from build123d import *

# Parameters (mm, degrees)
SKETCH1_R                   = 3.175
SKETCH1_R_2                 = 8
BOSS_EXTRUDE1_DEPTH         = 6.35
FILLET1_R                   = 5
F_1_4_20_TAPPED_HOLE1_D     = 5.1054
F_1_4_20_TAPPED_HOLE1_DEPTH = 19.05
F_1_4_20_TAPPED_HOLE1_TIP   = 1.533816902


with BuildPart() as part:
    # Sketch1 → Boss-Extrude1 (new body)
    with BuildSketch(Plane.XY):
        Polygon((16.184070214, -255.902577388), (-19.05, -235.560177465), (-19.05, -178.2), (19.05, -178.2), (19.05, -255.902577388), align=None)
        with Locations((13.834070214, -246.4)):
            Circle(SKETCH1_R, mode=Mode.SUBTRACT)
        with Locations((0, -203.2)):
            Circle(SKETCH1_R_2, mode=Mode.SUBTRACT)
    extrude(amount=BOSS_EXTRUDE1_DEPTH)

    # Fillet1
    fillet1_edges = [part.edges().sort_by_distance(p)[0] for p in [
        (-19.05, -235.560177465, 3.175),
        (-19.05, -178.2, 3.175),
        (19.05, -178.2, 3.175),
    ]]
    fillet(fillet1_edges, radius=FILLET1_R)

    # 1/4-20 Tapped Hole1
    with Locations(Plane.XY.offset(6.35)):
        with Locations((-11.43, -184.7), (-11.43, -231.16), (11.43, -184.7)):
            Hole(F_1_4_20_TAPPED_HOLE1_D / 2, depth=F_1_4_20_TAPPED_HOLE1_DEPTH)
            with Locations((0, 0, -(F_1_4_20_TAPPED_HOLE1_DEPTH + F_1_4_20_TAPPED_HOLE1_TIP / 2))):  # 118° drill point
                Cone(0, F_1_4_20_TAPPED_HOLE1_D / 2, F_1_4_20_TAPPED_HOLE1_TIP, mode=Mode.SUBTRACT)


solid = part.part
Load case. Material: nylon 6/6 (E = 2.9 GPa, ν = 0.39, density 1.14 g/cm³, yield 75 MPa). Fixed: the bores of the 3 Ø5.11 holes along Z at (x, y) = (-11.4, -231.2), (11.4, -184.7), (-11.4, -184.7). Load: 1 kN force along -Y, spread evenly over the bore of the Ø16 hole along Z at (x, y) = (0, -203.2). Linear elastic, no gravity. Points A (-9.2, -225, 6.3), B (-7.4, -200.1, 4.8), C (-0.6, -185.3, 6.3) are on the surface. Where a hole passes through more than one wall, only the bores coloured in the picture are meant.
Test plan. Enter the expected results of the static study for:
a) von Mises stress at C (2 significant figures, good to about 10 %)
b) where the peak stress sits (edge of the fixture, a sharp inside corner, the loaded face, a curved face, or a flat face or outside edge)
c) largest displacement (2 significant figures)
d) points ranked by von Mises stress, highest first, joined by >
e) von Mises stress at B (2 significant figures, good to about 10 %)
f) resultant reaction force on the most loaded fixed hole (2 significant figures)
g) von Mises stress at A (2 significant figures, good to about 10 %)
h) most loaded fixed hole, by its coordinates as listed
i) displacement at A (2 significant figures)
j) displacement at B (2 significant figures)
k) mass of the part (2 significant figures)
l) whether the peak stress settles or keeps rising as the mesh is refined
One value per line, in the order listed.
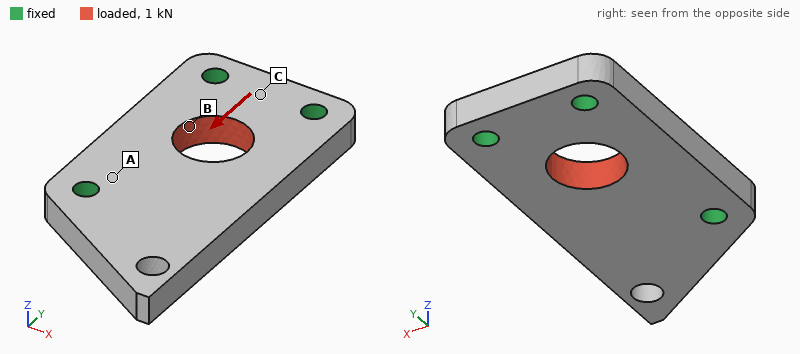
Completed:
1.1 MPa
edge of the fixture
41 µm
B > A > C
5.3 MPa
390 N
3.8 MPa
(11.4, -184.7)
7.3 µm
20 µm
17 g
keeps rising
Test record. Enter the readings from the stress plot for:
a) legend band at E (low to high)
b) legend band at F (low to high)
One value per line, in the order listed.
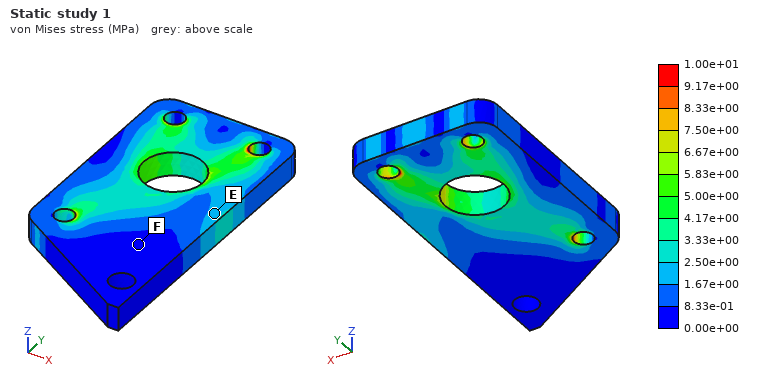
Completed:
1.67e+00 to 2.50e+00 MPa
0.00e+00 to 8.33e-01 MPa
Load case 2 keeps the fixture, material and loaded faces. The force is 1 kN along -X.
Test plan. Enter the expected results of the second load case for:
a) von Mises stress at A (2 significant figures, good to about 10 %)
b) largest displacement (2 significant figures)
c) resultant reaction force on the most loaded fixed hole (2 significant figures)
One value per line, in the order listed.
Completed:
4.5 MPa
71 µm
390 N
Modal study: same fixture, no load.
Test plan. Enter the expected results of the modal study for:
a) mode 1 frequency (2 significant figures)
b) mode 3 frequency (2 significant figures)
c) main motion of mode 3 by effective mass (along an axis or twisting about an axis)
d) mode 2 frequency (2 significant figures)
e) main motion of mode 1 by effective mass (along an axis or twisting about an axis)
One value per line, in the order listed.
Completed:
1600 Hz
5000 Hz
along Z
2900 Hz
along Z
